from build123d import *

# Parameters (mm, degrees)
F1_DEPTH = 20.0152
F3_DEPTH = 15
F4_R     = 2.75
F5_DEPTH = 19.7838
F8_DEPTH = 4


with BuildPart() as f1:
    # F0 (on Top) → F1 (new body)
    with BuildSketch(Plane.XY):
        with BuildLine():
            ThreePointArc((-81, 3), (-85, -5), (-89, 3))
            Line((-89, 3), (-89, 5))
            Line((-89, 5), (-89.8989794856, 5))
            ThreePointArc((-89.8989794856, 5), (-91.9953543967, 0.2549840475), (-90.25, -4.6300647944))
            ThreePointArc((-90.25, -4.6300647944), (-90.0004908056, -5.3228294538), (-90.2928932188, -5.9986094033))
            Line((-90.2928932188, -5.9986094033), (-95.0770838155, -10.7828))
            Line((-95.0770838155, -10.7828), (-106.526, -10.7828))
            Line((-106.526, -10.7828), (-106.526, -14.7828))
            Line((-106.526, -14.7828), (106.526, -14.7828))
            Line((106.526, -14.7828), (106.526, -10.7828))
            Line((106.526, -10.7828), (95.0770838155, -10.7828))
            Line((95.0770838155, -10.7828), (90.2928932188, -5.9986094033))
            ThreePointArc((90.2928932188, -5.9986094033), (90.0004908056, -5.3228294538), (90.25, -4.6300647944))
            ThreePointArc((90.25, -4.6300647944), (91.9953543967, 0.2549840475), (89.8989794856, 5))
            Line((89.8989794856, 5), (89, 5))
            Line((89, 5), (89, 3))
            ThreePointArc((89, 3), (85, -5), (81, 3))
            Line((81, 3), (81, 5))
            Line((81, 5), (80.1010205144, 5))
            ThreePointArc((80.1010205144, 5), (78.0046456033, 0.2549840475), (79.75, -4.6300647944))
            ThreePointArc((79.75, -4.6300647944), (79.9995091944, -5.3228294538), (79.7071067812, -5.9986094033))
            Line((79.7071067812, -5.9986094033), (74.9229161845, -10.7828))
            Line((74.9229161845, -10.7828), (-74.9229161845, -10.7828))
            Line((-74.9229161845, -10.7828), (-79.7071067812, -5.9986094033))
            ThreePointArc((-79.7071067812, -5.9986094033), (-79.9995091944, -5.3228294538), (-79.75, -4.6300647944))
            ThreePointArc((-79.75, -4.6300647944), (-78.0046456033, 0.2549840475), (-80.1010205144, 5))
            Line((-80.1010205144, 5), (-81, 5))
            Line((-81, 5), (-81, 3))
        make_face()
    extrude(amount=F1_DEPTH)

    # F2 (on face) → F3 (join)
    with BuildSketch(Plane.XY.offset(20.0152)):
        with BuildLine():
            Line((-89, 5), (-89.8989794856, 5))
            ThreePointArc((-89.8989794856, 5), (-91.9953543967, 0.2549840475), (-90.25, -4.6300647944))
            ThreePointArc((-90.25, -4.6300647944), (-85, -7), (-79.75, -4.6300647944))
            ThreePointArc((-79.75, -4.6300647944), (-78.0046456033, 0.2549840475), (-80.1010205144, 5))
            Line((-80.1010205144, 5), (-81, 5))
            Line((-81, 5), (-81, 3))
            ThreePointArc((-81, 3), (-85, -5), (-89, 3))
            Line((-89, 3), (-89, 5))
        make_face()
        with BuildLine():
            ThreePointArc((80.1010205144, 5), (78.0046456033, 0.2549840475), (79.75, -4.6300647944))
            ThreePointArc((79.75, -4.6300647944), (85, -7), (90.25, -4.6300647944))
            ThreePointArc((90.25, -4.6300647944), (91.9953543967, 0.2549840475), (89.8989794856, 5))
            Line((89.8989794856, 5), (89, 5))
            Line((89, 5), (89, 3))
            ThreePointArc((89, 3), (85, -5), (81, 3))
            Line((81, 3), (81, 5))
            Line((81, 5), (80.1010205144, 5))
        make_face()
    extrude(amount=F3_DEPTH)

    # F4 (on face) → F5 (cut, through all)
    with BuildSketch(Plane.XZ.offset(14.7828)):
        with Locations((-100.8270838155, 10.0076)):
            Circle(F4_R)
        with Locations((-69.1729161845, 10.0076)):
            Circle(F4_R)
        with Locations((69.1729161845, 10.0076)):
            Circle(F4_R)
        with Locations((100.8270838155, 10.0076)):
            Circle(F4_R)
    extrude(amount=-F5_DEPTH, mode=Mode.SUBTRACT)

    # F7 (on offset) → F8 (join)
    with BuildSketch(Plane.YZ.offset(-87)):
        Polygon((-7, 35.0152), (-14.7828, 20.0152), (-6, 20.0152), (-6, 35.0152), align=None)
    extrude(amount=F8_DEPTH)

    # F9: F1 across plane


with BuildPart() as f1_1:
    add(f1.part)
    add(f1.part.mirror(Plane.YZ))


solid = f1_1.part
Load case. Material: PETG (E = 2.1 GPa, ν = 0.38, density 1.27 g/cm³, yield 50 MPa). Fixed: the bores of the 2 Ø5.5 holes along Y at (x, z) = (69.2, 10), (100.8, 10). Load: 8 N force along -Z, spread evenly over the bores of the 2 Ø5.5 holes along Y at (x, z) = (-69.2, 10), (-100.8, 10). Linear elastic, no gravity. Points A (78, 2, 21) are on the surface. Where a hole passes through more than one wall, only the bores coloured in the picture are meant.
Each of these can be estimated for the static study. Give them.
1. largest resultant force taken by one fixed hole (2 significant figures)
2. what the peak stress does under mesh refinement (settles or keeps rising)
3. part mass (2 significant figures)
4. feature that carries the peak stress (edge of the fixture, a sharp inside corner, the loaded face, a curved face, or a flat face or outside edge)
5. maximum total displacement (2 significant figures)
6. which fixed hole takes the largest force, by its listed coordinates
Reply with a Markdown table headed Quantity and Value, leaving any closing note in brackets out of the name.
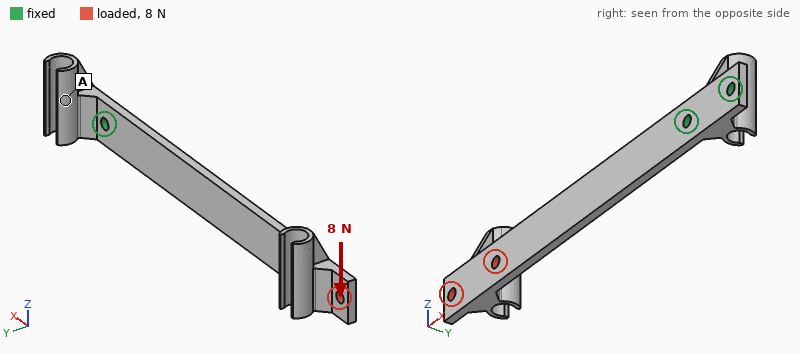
| Quantity | Value |
|---|---|
| largest resultant force taken by one fixed hole | 32 N |
| what the peak stress does under mesh refinement | keeps rising |
| part mass | 30 g |
| feature that carries the peak stress | edge of the fixture |
| maximum total displacement | 2.4 mm |
| which fixed hole takes the largest force, by its listed coordinates | (69.2, 10) |
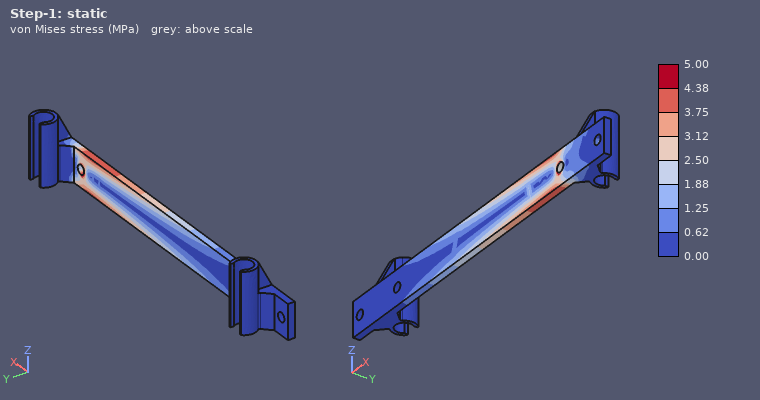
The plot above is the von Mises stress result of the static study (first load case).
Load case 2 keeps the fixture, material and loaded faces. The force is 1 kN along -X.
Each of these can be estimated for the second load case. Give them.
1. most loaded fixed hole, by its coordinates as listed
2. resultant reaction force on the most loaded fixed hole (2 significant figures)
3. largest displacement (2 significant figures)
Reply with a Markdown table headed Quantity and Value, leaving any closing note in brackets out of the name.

| Quantity | Value |
|---|---|
| most loaded fixed hole, by its coordinates as listed | (69.2, 10) |
| resultant reaction force on the most loaded fixed hole | 900 N |
| largest displacement | 1.0 mm |
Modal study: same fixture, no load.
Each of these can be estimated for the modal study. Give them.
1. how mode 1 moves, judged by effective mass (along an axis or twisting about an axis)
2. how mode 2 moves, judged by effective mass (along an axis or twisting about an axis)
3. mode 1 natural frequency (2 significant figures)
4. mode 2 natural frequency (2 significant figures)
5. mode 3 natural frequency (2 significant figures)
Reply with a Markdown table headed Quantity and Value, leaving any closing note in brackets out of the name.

| Quantity | Value |
|---|---|
| how mode 1 moves, judged by effective mass | along Y |
| how mode 2 moves, judged by effective mass | along Z |
| mode 1 natural frequency | 21 Hz |
| mode 2 natural frequency | 95 Hz |
| mode 3 natural frequency | 160 Hz |
